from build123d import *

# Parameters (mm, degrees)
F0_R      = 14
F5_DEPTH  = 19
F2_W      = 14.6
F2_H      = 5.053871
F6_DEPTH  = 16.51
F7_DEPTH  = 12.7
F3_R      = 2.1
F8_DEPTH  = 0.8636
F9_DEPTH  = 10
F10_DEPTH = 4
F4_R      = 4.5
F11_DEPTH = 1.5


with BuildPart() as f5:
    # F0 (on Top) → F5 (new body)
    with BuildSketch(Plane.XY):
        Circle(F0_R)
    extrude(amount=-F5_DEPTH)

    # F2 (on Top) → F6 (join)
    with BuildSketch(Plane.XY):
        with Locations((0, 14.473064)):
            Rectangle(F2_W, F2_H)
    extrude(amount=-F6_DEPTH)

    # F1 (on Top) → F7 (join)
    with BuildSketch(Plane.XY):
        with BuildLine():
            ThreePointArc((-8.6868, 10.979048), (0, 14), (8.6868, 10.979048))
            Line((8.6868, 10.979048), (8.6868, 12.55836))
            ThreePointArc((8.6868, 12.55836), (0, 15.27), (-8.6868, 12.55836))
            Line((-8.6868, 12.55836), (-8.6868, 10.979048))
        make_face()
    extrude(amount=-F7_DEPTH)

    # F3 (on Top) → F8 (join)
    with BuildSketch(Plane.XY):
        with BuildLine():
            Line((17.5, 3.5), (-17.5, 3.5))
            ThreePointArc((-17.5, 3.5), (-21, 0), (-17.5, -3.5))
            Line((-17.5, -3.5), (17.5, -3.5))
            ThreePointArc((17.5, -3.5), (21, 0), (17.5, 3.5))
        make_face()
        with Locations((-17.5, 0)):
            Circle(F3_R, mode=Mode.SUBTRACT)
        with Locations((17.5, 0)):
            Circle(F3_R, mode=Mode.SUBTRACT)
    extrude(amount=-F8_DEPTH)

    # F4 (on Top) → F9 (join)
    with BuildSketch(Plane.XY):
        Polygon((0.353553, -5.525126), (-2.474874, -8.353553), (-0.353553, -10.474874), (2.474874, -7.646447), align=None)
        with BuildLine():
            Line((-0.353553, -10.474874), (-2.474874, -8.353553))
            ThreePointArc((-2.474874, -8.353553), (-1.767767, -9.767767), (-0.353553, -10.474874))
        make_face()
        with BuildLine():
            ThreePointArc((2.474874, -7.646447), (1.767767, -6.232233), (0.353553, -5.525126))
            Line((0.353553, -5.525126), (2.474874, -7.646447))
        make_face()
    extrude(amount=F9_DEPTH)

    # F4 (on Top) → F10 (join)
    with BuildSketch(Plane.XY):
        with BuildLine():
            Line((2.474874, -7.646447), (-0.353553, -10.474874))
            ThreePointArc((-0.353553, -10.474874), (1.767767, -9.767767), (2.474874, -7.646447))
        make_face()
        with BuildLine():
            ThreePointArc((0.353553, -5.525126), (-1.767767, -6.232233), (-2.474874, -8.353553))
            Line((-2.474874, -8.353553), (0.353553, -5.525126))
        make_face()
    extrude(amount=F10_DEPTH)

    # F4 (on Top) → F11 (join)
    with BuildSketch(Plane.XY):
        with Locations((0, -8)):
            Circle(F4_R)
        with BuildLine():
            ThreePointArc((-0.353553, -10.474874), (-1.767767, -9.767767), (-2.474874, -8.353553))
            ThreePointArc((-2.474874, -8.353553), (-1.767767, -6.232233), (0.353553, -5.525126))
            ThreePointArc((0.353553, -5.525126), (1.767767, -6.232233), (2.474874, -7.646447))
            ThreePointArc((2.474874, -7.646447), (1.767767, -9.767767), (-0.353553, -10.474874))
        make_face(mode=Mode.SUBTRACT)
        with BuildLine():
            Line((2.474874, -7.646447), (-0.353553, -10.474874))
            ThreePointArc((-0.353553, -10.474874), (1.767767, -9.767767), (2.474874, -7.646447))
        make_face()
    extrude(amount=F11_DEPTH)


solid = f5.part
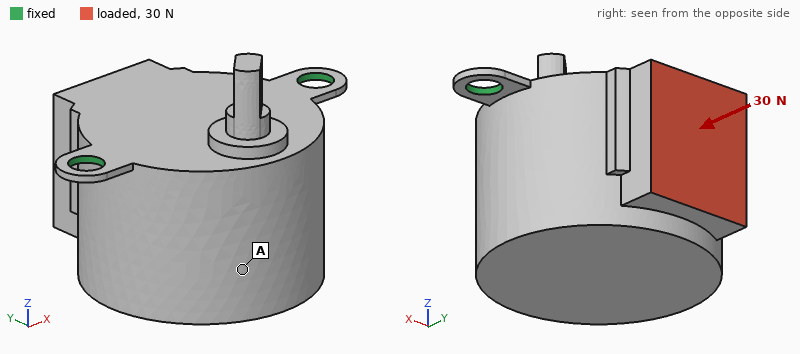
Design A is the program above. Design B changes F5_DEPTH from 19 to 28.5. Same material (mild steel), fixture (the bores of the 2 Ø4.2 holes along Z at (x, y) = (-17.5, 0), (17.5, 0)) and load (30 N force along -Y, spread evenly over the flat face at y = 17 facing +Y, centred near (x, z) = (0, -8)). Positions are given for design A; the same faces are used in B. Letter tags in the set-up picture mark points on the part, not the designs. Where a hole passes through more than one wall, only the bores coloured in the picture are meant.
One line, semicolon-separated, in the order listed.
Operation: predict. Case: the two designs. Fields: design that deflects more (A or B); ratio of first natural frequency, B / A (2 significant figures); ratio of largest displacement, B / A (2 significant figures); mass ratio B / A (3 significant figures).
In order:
B; 0.62; 1.3; 1.45
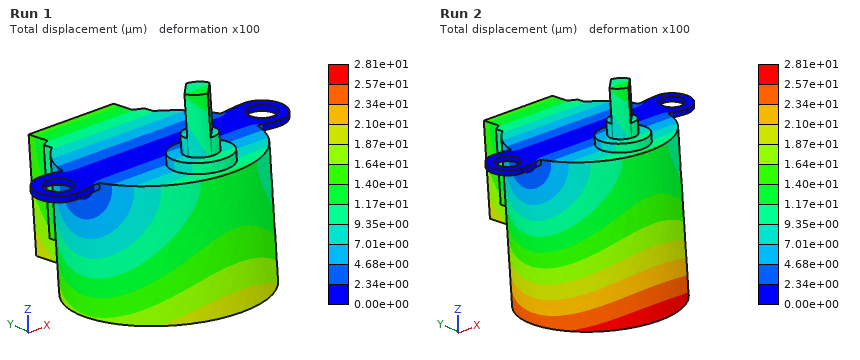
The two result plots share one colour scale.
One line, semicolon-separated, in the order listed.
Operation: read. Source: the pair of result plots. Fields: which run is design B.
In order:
Run 2
